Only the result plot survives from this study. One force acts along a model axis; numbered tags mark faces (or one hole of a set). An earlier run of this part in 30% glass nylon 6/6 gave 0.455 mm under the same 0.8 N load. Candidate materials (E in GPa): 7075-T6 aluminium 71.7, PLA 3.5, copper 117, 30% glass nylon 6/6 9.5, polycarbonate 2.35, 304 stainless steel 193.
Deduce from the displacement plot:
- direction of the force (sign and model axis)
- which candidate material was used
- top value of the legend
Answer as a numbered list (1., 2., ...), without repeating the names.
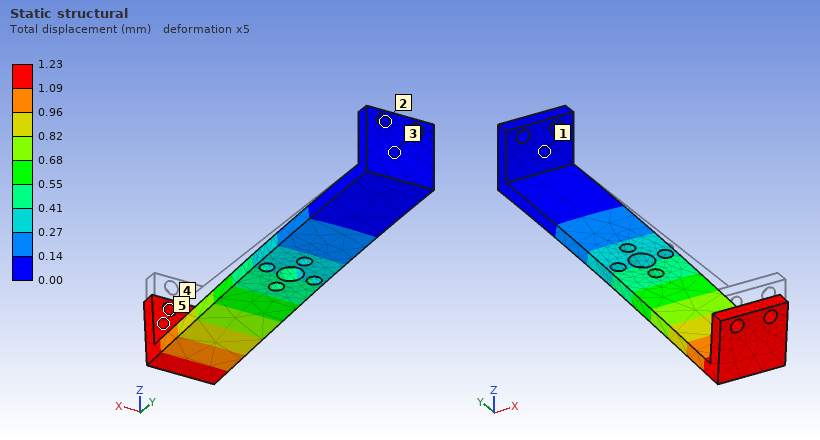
1. -Z
2. PLA
3. 1.23 mm
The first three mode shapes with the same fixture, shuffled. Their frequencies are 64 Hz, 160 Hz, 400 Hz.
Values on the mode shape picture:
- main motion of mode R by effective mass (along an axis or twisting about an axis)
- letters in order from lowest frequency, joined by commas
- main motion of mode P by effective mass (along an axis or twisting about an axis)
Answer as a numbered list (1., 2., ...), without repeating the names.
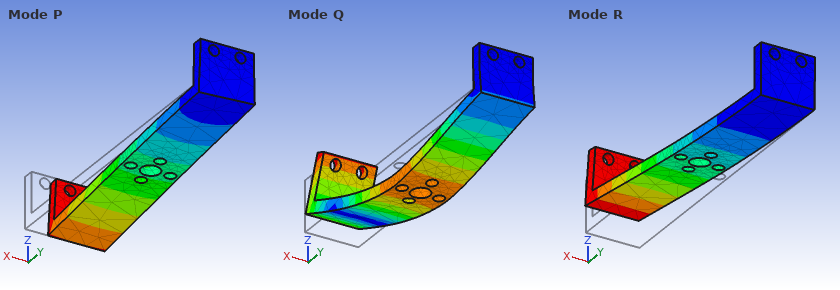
1. along Z
2. R, P, Q
3. along X
